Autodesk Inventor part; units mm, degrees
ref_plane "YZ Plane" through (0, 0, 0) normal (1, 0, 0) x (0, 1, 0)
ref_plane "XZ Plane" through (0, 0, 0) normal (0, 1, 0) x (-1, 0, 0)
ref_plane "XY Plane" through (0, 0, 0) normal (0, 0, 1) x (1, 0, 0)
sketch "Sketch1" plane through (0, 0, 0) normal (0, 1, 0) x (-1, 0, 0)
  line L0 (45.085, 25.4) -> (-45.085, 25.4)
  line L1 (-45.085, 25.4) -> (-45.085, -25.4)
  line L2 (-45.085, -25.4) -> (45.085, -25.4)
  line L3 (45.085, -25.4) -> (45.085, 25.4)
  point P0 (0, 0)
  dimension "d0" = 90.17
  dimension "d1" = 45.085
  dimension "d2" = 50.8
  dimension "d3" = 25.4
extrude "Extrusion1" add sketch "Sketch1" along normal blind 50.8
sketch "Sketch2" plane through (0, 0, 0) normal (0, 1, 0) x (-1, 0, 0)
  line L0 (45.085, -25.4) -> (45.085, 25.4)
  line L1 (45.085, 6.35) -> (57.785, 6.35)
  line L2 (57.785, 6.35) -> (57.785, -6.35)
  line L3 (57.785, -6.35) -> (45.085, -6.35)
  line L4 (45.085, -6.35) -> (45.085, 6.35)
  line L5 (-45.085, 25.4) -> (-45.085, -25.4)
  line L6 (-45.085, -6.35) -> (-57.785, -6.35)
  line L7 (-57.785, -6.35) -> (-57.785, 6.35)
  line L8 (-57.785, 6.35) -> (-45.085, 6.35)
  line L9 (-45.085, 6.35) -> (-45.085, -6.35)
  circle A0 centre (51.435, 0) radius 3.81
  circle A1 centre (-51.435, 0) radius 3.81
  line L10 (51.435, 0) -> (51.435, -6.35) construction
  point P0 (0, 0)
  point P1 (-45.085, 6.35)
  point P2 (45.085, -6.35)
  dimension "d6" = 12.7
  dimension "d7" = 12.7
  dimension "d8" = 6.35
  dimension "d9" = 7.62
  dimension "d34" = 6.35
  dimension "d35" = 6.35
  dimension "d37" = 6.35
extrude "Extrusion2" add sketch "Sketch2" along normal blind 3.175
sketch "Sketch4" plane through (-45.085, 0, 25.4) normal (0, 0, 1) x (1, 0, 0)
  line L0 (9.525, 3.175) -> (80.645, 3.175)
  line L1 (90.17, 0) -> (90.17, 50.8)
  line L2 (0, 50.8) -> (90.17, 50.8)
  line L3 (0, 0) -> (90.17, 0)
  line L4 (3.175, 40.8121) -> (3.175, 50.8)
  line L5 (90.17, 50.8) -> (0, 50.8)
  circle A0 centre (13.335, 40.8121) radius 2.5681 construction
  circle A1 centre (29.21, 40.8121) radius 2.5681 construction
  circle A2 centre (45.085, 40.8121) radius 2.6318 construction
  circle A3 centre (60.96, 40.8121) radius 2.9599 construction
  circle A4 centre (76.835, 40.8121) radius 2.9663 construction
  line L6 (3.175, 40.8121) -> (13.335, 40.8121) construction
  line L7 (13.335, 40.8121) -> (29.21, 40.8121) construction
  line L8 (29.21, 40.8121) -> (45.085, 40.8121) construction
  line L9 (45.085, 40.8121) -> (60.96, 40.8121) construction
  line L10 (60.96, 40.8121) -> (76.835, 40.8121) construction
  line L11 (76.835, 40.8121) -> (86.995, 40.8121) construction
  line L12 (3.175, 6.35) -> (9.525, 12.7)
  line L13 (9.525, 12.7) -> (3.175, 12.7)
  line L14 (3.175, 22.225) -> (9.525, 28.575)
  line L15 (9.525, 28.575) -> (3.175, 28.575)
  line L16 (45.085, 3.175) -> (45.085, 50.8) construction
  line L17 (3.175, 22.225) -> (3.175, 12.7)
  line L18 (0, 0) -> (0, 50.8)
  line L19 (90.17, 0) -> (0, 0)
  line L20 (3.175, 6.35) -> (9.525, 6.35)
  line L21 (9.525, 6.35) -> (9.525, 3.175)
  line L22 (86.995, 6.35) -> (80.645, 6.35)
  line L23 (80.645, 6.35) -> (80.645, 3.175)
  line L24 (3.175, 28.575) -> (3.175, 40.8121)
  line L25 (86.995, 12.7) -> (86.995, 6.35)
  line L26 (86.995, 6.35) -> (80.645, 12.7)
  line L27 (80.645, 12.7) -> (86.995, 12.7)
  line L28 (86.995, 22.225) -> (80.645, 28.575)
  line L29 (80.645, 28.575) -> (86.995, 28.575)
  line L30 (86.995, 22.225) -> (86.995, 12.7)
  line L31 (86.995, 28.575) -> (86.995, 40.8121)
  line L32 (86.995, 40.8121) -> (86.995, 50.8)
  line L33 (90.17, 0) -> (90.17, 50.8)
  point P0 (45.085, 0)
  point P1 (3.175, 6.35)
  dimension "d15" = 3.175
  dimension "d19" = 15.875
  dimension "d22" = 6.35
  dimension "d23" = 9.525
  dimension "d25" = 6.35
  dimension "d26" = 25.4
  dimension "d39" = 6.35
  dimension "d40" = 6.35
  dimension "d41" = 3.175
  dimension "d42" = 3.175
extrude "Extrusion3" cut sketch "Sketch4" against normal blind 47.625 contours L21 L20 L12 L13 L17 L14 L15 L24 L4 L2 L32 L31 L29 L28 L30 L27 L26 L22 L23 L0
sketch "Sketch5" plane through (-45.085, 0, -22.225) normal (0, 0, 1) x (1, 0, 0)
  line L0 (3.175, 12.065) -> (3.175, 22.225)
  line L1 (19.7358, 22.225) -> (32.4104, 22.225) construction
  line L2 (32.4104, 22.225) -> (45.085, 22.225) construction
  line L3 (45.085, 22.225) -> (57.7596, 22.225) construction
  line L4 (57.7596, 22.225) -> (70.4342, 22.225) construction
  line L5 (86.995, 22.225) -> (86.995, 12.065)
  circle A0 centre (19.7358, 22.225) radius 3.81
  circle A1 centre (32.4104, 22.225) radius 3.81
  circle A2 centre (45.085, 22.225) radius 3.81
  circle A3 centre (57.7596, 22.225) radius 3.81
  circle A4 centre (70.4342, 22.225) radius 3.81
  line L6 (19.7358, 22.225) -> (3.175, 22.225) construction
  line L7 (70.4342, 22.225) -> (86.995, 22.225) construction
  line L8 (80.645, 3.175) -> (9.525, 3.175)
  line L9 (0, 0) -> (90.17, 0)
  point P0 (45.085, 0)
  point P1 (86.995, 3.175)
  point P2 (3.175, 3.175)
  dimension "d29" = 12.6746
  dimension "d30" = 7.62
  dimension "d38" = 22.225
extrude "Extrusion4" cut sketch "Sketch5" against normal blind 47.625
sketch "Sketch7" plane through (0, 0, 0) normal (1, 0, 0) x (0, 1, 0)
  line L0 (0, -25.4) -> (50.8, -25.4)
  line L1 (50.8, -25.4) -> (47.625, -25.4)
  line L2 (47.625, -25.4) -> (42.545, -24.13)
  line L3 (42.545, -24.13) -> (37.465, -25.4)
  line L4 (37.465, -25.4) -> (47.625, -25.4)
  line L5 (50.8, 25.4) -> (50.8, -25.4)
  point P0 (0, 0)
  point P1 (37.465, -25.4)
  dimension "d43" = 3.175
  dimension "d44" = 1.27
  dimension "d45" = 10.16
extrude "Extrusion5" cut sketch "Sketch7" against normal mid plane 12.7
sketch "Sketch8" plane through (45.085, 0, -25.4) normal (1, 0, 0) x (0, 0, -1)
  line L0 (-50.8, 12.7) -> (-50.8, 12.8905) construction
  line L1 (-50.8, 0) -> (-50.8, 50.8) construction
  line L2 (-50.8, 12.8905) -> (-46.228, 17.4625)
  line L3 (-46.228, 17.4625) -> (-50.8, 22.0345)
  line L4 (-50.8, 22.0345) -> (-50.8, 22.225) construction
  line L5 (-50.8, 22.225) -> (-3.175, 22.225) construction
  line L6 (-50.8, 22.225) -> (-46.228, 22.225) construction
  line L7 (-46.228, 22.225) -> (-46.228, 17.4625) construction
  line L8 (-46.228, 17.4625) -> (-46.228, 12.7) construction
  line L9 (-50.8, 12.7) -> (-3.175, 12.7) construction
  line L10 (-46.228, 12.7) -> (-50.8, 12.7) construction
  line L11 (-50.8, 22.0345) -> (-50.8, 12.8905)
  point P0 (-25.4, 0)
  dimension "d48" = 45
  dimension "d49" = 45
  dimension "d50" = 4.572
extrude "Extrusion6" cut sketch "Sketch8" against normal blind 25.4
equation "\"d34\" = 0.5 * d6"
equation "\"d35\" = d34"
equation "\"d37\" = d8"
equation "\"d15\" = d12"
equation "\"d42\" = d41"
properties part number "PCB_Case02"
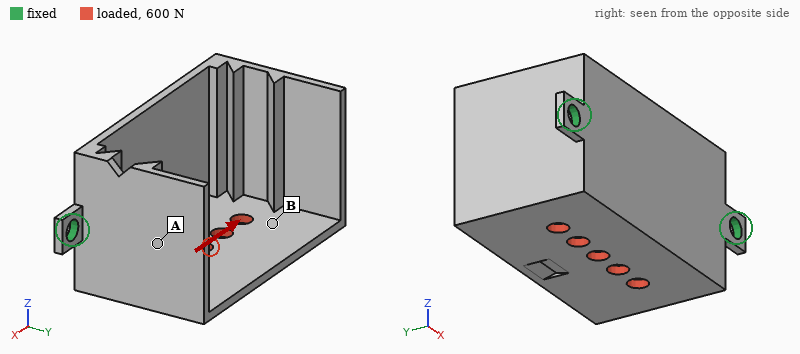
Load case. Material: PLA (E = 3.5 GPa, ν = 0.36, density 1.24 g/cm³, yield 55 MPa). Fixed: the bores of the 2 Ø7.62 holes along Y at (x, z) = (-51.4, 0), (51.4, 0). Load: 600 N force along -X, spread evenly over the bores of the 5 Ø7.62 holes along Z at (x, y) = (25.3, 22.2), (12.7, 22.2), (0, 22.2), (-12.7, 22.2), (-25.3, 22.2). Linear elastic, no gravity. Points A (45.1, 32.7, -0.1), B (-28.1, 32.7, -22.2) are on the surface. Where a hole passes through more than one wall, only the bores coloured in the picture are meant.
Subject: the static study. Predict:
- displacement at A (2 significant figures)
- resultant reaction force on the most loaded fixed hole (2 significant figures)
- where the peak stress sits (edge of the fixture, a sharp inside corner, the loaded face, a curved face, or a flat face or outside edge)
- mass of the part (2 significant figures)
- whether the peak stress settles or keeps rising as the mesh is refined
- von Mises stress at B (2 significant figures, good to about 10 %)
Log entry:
0.81 mm
360 N
edge of the fixture
60 g
keeps rising
6.9 MPa
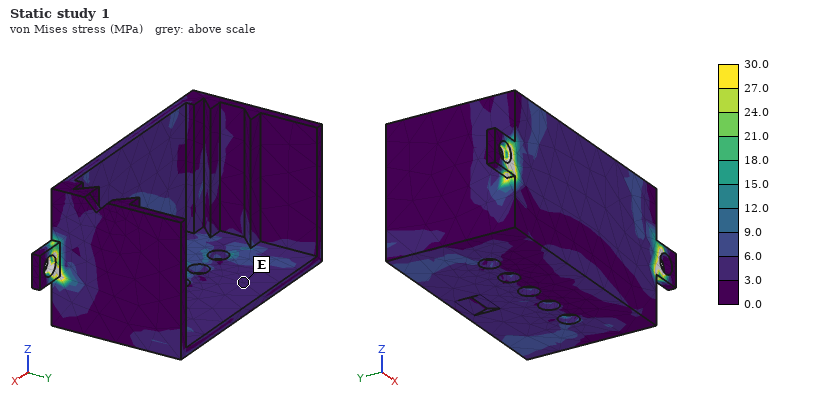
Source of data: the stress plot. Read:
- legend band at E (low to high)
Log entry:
3.0 to 6.0 MPa
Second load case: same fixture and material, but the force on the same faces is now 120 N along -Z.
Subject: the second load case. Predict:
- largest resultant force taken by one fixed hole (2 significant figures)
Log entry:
61 N
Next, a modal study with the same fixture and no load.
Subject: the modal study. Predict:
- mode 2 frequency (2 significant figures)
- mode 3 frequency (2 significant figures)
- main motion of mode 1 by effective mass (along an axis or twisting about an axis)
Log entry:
400 Hz
590 Hz
along Z
